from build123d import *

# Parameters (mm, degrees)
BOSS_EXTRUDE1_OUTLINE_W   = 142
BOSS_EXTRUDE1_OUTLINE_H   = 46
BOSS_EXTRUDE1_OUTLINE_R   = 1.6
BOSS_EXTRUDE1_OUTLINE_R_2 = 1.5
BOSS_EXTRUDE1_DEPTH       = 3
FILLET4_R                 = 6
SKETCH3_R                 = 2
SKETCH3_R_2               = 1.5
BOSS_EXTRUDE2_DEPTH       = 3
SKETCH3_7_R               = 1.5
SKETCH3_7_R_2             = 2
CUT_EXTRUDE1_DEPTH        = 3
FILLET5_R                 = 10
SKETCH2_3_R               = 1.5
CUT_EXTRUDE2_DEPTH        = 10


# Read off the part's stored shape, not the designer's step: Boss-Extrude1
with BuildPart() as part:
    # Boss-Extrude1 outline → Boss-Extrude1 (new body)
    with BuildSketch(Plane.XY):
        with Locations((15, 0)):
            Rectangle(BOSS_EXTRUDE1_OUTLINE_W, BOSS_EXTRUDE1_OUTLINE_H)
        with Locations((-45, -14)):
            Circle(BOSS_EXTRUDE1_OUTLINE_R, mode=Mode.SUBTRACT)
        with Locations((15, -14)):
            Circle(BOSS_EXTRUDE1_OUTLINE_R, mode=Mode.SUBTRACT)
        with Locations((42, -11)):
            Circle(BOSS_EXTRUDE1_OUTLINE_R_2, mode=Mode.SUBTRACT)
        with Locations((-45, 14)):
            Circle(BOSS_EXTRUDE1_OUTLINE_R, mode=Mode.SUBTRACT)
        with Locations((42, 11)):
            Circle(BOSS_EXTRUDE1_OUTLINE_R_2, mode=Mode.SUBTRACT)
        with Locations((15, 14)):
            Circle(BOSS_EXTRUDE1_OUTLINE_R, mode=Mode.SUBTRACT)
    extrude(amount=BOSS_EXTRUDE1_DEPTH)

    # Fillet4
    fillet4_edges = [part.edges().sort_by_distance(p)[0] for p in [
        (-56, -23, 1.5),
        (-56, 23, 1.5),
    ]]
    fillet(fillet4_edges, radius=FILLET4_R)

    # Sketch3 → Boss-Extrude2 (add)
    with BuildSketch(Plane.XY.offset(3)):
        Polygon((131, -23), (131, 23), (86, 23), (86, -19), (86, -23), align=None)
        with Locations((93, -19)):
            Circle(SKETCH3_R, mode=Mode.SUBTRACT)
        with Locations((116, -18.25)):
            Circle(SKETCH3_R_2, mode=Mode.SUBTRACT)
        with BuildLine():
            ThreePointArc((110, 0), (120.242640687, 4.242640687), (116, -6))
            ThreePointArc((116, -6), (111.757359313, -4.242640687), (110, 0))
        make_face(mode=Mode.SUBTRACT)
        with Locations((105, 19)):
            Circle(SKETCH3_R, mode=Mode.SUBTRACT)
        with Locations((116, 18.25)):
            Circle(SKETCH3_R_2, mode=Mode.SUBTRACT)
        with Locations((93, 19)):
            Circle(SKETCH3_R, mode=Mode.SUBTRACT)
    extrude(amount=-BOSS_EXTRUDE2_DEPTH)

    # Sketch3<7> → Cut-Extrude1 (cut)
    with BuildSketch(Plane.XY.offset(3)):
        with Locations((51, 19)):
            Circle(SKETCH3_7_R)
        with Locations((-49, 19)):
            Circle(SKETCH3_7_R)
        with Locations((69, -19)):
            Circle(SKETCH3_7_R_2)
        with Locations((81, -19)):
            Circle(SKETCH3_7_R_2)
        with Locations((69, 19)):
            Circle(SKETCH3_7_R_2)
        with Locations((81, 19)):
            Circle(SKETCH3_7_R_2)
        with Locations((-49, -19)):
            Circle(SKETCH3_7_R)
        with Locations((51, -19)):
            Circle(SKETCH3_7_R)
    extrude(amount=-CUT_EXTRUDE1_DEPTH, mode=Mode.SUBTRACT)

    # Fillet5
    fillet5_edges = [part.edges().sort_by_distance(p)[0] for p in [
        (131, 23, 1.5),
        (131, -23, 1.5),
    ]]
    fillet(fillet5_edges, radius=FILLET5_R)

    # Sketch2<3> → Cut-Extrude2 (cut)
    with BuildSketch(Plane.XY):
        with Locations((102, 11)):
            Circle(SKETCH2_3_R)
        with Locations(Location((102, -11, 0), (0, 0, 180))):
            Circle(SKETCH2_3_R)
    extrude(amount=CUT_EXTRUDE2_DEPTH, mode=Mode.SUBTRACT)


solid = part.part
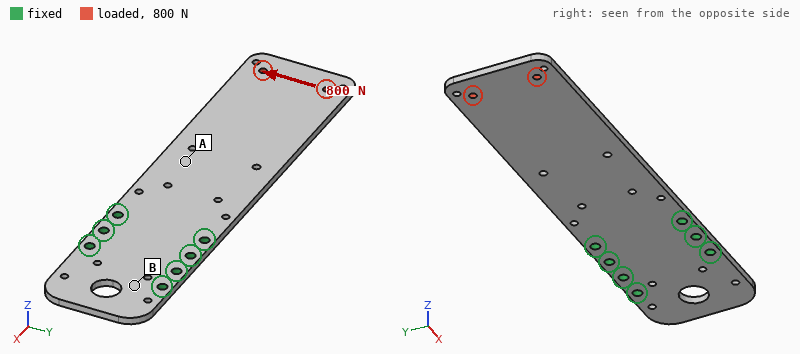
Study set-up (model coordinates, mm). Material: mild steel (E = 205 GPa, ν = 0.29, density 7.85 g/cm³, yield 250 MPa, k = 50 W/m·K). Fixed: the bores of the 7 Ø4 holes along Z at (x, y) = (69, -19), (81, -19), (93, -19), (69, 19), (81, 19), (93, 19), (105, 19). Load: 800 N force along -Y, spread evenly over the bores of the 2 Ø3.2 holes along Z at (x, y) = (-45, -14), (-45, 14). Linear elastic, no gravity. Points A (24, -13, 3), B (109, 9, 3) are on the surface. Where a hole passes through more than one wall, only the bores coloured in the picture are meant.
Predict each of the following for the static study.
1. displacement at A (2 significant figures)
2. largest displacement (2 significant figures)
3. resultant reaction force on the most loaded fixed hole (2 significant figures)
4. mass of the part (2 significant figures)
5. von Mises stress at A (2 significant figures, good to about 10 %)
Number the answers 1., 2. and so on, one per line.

1. 0.023 mm
2. 0.11 mm
3. 2.2 kN
4. 190 g
5. 29 MPa
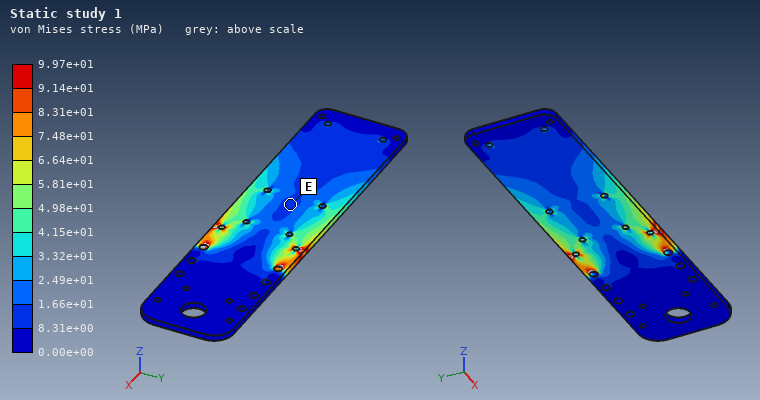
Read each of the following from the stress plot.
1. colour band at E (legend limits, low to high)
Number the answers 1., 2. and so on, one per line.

1. 8.31e+00 to 1.66e+01 MPa
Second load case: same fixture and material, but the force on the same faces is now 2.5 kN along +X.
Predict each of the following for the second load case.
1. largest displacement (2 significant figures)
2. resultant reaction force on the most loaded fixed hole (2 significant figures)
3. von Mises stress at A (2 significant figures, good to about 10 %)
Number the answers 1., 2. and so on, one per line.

1. 12 µm
2. 880 N
3. 17 MPa
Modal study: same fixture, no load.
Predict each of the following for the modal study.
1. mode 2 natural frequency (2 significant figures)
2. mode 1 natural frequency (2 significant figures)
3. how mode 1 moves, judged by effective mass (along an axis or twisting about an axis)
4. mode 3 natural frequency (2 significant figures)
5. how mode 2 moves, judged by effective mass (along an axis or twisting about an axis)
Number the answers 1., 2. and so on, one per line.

1. 910 Hz
2. 160 Hz
3. along Z
4. 990 Hz
5. twisting about X
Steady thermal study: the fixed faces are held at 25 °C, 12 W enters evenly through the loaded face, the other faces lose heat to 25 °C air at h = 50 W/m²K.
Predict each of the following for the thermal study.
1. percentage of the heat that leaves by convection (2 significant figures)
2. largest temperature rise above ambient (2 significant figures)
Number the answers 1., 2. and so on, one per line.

1. 94 %
2. 58 K
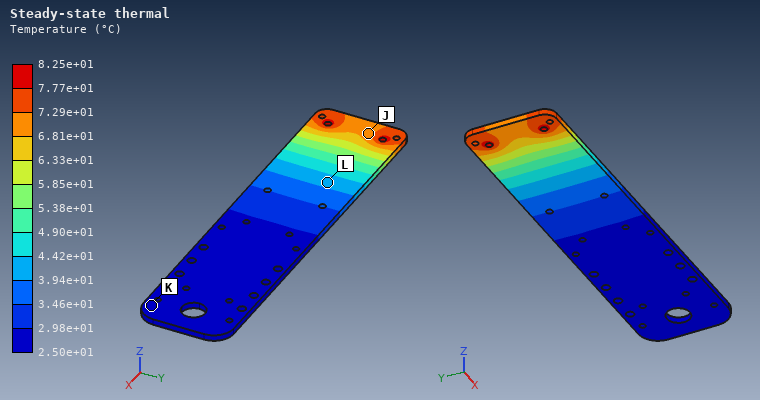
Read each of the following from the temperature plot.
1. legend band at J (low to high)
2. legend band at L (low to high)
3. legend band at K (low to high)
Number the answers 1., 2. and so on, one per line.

1. 6.81e+01 to 7.29e+01 °C
2. 3.94e+01 to 4.42e+01 °C
3. 2.50e+01 to 2.98e+01 °C
